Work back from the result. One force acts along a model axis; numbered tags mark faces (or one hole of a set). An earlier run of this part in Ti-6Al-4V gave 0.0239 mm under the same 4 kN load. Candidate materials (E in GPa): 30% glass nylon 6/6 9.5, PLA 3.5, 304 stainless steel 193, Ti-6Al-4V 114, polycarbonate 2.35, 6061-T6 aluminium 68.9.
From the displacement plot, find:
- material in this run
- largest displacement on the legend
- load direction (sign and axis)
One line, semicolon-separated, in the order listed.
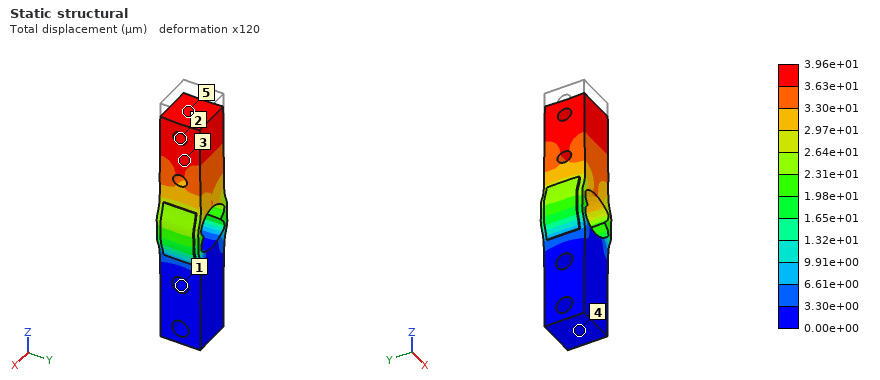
6061-T6 aluminium; 3.96e+01 µm; -Z
